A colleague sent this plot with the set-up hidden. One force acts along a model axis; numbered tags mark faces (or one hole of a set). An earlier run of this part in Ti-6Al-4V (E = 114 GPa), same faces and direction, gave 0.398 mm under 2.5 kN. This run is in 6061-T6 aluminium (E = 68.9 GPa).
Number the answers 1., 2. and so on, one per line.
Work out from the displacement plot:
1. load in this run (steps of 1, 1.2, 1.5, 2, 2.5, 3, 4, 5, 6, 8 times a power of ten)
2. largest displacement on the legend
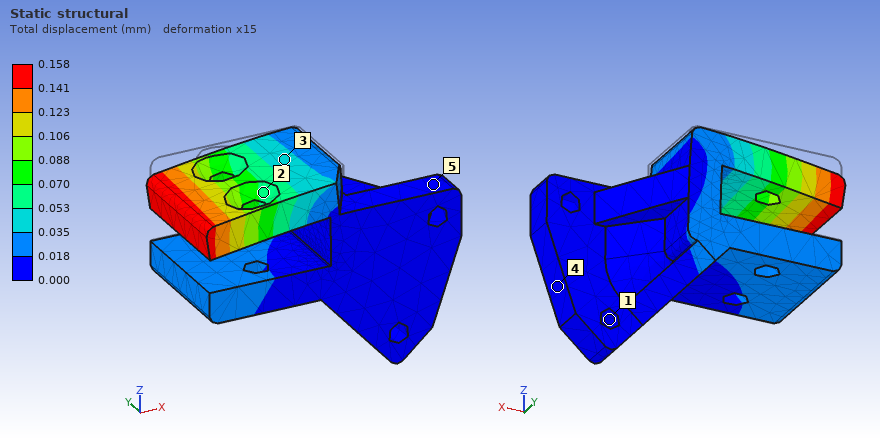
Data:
1. 600 N
2. 0.158 mm
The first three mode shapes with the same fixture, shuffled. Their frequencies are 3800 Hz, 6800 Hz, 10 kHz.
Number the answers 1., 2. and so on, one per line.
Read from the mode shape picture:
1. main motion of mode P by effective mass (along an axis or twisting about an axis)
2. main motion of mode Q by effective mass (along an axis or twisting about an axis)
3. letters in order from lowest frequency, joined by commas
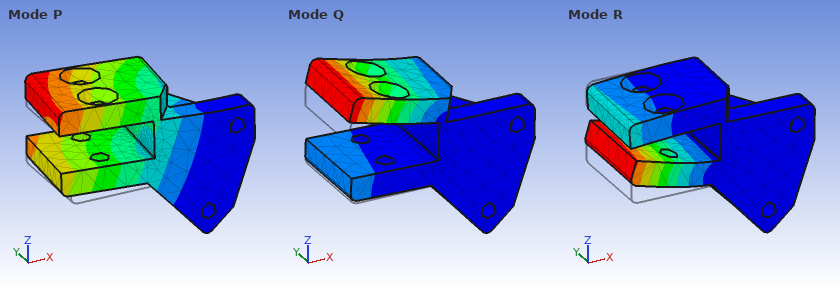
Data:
1. along Y
2. along Z
3. P, Q, R
